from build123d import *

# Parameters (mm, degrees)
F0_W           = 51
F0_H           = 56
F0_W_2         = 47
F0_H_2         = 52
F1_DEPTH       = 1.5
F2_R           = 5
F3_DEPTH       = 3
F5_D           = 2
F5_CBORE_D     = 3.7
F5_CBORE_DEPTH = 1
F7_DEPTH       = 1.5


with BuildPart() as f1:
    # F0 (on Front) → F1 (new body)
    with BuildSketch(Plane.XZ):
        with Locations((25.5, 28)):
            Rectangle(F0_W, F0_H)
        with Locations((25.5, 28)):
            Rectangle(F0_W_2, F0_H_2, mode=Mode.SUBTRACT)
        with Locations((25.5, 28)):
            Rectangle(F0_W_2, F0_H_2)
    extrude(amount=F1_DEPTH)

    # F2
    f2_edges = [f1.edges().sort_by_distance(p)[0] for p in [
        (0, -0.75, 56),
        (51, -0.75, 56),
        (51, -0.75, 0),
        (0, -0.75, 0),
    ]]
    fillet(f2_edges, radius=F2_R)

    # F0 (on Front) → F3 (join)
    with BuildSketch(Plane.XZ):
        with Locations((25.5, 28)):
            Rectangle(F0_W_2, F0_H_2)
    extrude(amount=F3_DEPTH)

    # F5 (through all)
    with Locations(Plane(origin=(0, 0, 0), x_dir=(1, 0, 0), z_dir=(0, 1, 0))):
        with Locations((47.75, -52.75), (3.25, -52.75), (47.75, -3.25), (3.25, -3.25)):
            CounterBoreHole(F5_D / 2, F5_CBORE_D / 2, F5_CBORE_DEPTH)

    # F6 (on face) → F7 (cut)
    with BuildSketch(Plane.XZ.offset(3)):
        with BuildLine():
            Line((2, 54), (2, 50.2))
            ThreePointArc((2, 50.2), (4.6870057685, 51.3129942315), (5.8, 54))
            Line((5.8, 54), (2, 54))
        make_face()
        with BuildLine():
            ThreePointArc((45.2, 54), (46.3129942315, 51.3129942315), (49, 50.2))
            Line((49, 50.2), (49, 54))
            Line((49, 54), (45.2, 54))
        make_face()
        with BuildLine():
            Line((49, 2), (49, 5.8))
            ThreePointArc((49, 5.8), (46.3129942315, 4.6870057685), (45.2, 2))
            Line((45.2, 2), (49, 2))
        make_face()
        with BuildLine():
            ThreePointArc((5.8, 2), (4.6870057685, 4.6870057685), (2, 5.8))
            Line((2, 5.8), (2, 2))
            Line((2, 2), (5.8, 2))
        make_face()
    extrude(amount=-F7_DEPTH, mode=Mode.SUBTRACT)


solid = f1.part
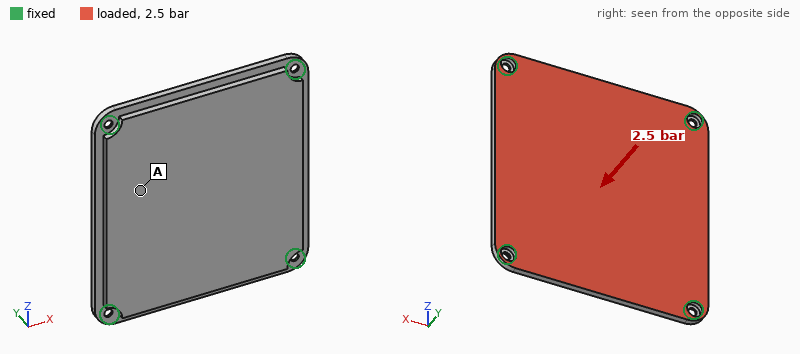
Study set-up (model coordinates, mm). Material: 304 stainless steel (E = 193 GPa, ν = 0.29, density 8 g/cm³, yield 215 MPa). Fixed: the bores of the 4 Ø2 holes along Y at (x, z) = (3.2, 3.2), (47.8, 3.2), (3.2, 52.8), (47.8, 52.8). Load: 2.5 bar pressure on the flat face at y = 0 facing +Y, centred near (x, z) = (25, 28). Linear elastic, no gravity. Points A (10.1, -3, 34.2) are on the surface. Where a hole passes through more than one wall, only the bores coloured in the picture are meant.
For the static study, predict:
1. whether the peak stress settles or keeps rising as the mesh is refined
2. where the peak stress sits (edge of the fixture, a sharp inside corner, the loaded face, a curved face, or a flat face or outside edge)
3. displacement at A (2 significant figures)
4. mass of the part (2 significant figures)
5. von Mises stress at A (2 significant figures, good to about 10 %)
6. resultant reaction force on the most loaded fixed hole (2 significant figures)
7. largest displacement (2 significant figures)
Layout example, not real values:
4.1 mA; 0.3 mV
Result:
keeps rising; edge of the fixture; 45 µm; 62 g; 41 MPa; 210 N; 55 µm
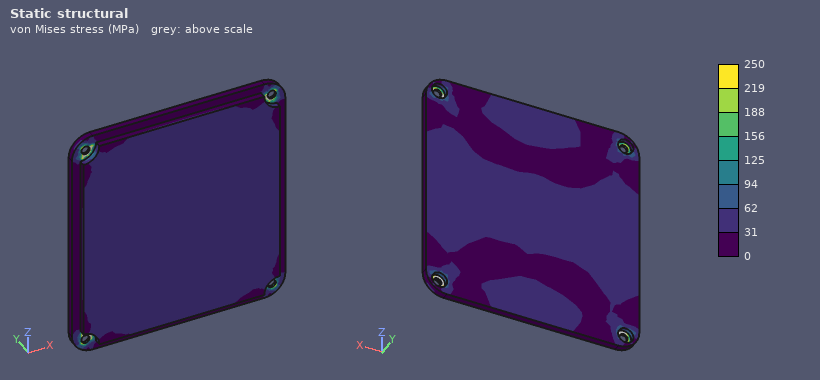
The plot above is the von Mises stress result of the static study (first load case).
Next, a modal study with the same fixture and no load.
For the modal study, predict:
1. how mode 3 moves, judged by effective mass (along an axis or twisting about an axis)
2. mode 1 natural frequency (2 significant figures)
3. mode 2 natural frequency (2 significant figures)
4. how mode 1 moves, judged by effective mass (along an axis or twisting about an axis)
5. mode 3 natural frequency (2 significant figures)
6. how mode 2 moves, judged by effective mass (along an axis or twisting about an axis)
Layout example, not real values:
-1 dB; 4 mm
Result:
twisting about X; 2600 Hz; 4800 Hz; along Y; 5300 Hz; twisting about Z
